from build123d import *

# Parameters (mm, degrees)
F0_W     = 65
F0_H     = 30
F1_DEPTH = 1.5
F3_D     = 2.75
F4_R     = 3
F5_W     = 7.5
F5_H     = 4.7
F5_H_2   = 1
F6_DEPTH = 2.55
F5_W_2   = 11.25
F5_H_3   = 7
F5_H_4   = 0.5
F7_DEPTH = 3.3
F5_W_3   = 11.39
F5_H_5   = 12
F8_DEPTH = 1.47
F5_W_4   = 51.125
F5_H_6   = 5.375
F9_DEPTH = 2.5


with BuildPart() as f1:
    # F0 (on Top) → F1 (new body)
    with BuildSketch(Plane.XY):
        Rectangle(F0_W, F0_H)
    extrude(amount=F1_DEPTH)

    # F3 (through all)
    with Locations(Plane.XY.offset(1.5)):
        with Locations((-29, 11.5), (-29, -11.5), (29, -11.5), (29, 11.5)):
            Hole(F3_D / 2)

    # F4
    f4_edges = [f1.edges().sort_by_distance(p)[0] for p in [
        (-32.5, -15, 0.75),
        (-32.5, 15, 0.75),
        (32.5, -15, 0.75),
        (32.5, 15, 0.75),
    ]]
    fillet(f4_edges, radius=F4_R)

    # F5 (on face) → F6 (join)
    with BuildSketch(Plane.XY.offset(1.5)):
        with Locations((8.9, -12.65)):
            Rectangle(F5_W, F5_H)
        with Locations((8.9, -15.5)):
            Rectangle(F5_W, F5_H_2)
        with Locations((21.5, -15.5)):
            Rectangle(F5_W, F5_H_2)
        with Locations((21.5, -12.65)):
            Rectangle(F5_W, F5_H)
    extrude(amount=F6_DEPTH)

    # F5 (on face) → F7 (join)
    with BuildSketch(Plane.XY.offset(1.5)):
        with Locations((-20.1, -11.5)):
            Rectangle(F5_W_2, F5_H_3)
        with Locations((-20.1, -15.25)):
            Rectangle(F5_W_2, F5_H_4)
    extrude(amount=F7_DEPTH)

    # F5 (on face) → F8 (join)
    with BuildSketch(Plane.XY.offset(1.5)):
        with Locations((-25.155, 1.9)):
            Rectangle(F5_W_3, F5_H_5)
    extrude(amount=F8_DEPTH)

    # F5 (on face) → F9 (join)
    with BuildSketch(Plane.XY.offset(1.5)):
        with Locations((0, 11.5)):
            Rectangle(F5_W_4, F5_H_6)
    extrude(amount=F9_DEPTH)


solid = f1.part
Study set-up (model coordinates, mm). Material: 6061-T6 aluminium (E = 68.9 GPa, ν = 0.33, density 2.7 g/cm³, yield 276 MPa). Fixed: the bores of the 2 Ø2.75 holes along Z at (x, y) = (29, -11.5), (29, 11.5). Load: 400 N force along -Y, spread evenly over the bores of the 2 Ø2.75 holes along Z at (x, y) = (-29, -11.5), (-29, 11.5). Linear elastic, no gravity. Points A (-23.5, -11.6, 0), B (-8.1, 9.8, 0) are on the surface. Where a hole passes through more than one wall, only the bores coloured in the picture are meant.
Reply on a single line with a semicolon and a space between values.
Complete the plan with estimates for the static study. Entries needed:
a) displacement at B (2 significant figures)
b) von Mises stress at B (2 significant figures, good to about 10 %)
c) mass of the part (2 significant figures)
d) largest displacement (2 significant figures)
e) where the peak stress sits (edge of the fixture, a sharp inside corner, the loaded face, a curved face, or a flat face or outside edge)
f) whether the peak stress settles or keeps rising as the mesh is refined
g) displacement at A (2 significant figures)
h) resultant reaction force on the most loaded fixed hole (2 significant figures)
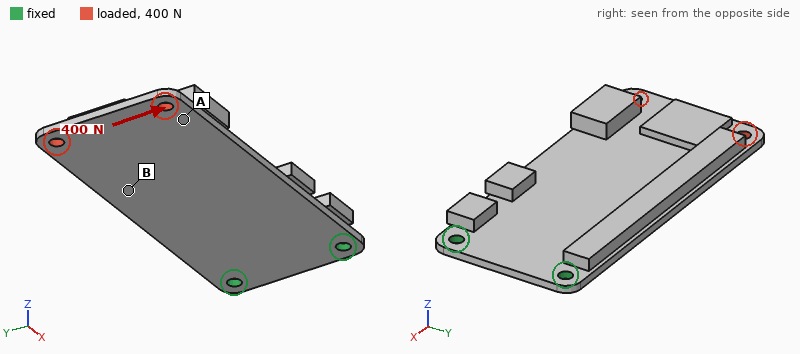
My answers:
0.11 mm; 29 MPa; 12 g; 0.31 mm; edge of the fixture; keeps rising; 0.24 mm; 1000 N
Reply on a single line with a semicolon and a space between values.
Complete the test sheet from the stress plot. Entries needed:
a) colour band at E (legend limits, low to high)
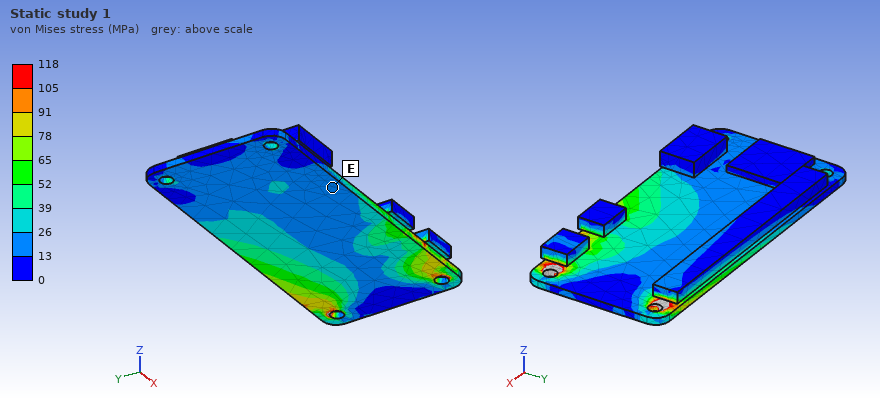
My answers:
13 to 26 MPa
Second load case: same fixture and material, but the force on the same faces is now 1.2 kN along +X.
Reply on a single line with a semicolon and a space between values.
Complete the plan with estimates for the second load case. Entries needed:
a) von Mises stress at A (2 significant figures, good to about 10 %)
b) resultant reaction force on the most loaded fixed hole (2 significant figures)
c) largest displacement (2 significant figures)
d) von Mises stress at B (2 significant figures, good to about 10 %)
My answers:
44 MPa; 610 N; 0.23 mm; 31 MPa
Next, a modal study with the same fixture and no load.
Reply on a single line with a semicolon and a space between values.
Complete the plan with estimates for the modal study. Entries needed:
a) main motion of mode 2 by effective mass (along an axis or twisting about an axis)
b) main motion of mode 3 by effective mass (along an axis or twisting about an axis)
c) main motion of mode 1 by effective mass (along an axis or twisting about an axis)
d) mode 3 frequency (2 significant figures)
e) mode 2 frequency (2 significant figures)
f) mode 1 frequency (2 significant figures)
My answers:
twisting about X; along Z; along Z; 2900 Hz; 1700 Hz; 380 Hz
